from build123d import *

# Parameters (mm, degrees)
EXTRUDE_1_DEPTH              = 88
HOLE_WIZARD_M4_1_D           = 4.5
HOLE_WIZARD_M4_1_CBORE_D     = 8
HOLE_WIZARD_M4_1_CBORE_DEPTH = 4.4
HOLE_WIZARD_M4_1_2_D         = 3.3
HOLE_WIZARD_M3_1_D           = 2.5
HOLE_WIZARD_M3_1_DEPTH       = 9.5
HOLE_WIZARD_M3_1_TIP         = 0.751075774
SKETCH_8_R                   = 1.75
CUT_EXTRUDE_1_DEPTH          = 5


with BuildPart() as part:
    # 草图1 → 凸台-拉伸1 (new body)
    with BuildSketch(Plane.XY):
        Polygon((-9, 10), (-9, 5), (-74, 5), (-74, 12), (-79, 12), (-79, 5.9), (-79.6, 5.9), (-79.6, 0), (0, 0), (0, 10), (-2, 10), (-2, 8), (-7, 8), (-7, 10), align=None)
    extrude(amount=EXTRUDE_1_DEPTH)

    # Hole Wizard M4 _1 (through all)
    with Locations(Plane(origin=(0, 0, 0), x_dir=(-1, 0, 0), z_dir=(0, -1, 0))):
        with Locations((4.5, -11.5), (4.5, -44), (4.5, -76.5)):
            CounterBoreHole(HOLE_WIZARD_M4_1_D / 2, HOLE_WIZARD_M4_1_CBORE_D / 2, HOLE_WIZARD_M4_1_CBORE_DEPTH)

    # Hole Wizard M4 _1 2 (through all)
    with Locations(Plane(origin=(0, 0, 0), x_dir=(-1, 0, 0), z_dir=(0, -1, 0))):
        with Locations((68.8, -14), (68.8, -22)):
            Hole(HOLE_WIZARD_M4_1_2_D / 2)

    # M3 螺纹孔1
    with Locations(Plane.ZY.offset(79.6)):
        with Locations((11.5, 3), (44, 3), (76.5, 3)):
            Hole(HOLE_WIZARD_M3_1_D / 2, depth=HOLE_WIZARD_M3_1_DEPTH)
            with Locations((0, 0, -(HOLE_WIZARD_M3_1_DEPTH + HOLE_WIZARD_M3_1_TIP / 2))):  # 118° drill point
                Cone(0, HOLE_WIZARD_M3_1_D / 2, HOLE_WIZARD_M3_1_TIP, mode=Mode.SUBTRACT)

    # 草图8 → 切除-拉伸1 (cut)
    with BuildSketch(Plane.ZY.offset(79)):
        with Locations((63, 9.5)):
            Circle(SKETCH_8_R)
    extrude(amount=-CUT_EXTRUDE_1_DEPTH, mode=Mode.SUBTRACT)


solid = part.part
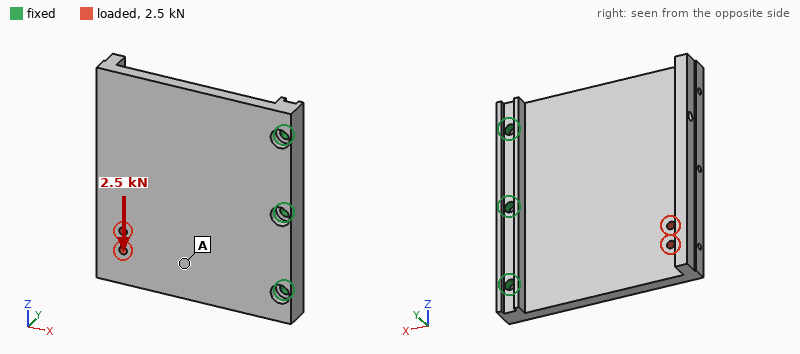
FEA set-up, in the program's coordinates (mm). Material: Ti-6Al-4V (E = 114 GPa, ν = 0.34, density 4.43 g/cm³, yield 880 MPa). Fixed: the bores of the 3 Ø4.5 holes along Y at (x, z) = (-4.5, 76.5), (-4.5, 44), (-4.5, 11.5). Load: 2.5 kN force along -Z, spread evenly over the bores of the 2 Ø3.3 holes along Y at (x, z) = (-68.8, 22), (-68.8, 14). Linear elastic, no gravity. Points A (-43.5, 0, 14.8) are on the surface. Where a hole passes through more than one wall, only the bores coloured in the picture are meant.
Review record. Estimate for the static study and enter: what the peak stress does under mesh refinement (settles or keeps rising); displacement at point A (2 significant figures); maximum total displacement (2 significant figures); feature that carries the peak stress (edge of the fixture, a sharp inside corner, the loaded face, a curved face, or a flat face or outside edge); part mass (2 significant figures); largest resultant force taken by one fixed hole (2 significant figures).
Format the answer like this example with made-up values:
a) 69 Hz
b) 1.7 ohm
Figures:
a) keeps rising
b) 29 µm
c) 62 µm
d) edge of the fixture
e) 180 g
f) 2.5 kN
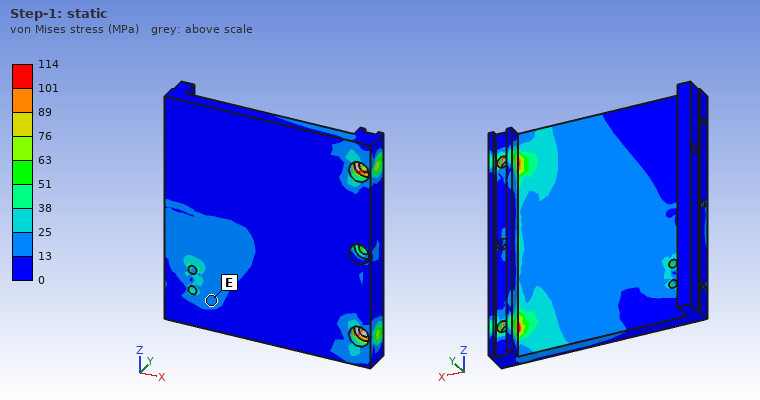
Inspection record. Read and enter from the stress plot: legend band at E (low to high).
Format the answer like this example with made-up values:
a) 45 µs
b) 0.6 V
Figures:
a) 13 to 25 MPa
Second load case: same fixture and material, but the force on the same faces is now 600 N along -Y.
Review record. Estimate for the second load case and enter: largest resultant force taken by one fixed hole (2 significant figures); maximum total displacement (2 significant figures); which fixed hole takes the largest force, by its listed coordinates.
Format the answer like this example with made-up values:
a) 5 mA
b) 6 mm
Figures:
a) 450 N
b) 0.96 mm
c) (-4.5, 44)
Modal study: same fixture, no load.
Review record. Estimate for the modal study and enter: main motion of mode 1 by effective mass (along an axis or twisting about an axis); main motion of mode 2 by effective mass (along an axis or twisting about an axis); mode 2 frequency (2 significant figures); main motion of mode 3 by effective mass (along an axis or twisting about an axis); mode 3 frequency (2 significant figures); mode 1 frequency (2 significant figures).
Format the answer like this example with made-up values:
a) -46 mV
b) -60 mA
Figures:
a) along Y
b) twisting about X
c) 1400 Hz
d) along Y
e) 3700 Hz
f) 570 Hz
